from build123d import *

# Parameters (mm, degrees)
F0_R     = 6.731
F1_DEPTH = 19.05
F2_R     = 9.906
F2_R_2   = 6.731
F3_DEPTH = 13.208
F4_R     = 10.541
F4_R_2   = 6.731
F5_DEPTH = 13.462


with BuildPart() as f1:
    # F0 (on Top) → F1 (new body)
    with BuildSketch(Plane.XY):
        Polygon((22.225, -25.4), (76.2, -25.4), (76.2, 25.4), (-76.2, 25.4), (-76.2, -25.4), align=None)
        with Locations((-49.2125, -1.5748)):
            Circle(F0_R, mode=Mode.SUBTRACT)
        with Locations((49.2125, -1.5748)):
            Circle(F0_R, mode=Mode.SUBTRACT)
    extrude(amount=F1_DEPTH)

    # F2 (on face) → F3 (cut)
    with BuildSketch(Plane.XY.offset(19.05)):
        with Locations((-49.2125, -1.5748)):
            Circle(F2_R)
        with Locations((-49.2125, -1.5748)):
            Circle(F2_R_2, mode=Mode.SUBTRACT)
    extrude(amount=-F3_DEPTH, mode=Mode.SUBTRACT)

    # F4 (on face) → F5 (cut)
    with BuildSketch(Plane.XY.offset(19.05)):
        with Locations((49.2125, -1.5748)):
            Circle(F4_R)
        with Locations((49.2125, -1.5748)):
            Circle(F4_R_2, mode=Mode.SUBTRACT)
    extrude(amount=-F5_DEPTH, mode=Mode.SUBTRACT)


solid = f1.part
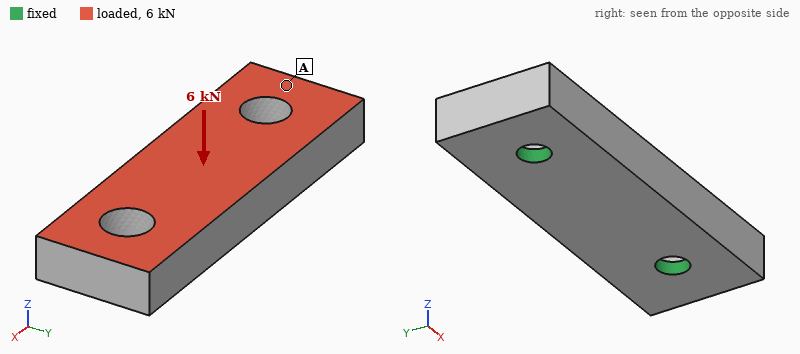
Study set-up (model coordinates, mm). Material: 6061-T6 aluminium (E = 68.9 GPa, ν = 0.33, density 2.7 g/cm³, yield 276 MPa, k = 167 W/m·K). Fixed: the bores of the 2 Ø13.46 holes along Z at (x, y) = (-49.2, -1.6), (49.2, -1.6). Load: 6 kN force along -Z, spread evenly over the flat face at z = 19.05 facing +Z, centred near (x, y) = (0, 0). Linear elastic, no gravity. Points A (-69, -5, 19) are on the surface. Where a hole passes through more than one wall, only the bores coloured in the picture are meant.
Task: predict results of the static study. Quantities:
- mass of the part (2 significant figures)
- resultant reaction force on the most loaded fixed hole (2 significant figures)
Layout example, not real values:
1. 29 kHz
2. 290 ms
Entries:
1. 370 g
2. 3.2 kN
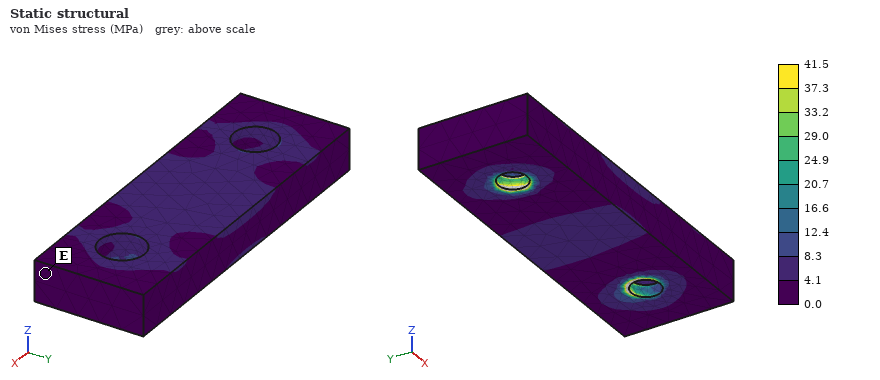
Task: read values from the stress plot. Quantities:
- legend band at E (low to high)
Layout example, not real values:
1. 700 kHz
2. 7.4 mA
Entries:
1. 0.0 to 4.1 MPa
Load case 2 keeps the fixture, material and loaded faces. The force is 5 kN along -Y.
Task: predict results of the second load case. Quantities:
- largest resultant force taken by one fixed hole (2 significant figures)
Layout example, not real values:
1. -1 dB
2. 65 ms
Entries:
1. 2.5 kN
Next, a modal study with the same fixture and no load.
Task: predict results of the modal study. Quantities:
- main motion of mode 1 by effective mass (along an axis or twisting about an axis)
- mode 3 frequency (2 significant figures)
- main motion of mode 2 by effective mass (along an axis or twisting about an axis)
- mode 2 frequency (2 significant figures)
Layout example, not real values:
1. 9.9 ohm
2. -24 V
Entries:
1. along Y
2. 7300 Hz
3. along Z
4. 5800 Hz
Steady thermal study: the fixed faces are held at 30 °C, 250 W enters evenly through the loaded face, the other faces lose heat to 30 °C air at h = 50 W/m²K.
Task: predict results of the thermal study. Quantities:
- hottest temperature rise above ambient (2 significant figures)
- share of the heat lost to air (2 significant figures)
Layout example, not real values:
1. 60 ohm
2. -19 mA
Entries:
1. 27 K
2. 6.1 %
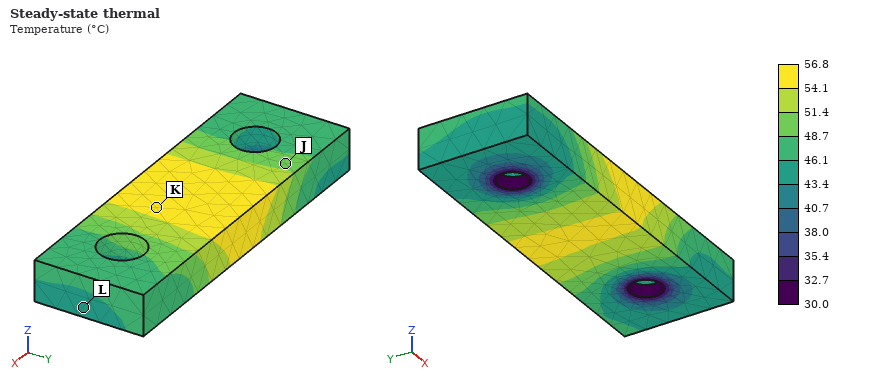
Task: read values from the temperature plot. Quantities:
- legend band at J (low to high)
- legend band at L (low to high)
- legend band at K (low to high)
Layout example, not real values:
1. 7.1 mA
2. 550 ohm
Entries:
1. 48.7 to 51.4 °C
2. 43.4 to 46.1 °C
3. 54.1 to 56.8 °C
